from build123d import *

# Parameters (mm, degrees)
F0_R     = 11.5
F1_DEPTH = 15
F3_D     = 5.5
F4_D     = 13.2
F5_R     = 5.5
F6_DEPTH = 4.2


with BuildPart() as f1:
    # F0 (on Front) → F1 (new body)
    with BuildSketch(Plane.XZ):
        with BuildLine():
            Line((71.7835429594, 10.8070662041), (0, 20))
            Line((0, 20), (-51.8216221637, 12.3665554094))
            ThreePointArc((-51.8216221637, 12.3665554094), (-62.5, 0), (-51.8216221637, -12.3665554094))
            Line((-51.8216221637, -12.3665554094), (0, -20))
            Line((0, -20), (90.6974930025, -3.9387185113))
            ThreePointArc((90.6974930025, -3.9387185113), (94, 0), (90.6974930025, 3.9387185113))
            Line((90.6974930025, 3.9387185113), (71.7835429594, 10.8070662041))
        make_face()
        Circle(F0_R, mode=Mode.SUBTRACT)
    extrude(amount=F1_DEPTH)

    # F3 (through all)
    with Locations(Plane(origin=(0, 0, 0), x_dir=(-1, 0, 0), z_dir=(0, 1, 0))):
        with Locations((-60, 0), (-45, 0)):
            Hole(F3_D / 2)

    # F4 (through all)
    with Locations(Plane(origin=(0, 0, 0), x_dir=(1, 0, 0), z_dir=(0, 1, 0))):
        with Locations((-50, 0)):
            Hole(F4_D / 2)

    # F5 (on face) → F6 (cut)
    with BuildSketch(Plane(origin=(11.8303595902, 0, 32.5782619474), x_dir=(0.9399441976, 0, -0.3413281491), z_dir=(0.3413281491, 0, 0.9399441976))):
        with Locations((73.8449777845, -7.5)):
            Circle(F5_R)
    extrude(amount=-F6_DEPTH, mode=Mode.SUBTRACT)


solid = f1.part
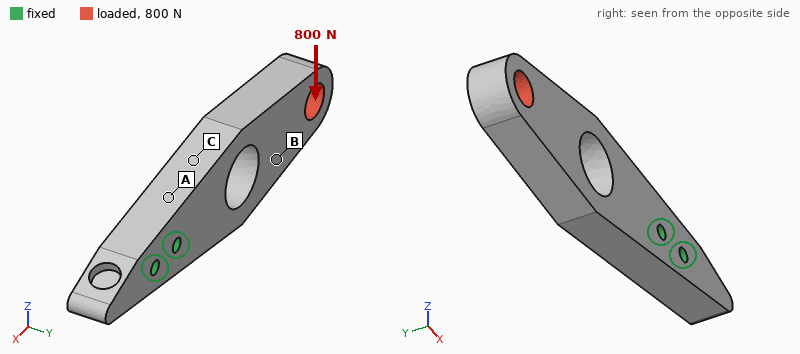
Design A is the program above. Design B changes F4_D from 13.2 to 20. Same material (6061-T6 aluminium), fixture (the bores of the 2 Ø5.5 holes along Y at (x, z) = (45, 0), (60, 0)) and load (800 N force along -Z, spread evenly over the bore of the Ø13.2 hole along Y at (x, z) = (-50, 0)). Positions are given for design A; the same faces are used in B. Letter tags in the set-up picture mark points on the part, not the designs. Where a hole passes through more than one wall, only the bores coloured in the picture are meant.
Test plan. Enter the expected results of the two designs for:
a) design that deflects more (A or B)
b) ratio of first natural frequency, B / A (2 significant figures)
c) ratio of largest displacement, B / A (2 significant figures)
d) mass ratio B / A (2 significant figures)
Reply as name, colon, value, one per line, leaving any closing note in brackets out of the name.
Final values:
design that deflects more: B
ratio of first natural frequency, B / A: 1.1
ratio of largest displacement, B / A: 1.1
mass ratio B / A: 0.95
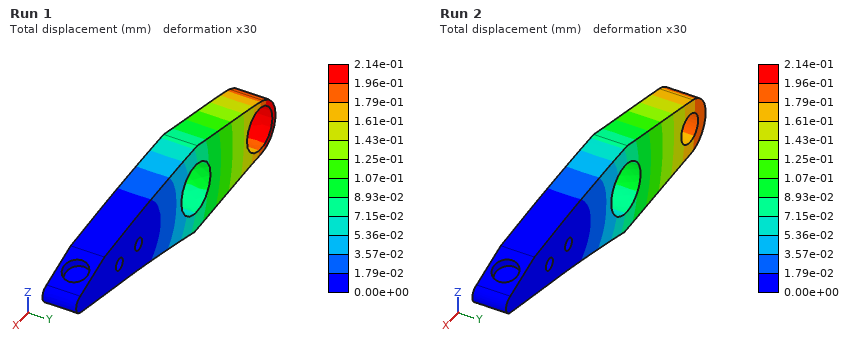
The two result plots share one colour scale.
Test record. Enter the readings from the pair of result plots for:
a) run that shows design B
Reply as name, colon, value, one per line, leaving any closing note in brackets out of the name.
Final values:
run that shows design B: Run 1
